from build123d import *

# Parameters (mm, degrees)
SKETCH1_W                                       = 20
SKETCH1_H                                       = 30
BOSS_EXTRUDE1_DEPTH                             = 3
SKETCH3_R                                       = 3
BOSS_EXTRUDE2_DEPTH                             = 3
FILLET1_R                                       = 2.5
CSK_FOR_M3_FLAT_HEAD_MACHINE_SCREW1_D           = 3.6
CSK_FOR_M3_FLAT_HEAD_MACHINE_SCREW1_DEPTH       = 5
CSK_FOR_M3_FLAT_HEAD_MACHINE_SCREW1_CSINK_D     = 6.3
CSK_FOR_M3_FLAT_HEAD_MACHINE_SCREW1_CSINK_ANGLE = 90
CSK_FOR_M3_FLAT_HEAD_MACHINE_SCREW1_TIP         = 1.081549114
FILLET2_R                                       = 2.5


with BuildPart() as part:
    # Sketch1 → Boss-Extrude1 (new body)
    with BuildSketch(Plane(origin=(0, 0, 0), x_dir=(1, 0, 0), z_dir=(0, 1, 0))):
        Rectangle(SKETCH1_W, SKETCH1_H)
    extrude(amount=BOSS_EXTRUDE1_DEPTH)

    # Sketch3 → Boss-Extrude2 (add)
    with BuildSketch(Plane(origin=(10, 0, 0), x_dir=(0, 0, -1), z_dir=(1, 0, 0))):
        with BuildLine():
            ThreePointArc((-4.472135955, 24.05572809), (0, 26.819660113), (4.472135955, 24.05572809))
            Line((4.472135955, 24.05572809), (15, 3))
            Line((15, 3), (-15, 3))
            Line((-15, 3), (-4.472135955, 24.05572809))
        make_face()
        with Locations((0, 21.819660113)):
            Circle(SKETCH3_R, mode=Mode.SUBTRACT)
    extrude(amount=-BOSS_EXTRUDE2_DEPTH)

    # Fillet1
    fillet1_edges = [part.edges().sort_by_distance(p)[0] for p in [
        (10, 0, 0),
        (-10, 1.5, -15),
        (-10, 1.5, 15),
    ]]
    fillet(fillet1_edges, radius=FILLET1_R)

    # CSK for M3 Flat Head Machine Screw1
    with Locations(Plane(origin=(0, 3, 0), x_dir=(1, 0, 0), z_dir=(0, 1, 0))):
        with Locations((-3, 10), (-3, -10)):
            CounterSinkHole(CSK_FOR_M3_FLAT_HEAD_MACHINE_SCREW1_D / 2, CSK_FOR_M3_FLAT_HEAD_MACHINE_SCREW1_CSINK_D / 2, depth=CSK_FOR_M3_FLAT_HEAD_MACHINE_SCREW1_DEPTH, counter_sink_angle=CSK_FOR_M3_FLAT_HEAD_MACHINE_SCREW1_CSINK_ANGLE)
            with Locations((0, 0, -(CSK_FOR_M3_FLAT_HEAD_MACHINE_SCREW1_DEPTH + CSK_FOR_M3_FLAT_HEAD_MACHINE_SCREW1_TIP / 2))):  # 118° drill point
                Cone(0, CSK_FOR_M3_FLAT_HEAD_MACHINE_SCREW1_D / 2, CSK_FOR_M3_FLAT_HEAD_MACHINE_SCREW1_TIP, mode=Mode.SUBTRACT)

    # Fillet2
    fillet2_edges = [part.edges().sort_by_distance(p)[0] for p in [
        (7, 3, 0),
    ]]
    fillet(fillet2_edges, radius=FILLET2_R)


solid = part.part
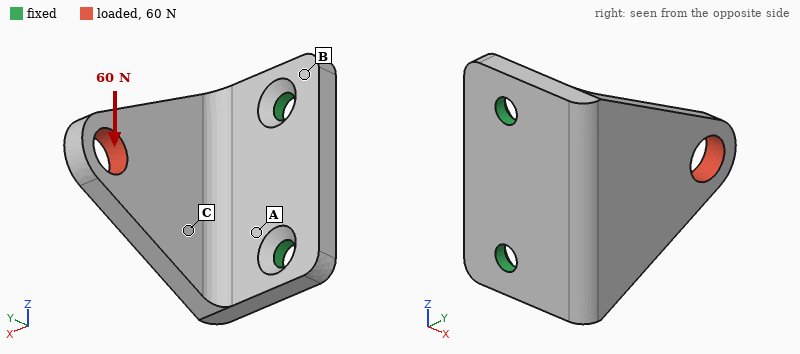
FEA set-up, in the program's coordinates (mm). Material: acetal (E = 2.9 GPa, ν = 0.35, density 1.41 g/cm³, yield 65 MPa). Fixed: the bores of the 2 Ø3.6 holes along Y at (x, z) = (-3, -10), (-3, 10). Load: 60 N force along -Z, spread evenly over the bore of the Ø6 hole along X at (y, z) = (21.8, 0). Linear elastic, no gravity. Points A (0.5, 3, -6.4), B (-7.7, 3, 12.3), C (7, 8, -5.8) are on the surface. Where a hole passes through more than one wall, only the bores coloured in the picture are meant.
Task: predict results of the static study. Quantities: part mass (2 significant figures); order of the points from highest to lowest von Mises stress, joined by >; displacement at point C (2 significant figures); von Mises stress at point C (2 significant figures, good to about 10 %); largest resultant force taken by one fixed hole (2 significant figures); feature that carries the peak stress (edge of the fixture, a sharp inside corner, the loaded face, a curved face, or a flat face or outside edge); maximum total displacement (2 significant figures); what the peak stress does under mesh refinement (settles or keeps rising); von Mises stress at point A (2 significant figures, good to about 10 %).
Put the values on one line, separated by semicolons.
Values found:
4.1 g; A > C > B; 0.15 mm; 6.7 MPa; 73 N; edge of the fixture; 0.47 mm; keeps rising; 12 MPa
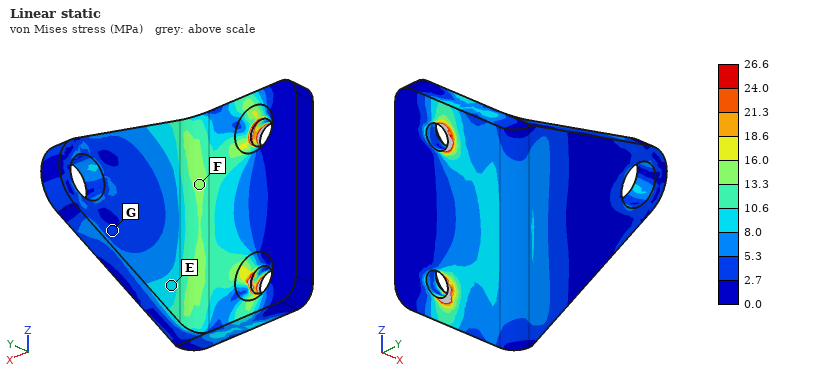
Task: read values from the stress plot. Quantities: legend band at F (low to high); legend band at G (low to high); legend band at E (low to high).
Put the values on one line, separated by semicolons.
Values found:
13.3 to 16.0 MPa; 2.7 to 5.3 MPa; 8.0 to 10.6 MPa
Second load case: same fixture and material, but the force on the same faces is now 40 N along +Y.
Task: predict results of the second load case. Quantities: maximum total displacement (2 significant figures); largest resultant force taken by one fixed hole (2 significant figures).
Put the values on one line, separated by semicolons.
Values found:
0.49 mm; 20 N
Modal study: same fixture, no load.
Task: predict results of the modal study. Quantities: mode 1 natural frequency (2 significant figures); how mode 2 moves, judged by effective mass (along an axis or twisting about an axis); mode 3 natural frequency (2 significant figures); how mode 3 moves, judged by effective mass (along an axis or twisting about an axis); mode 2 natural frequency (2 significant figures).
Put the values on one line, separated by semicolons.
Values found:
1000 Hz; along Z; 2800 Hz; along Y; 2300 Hz
